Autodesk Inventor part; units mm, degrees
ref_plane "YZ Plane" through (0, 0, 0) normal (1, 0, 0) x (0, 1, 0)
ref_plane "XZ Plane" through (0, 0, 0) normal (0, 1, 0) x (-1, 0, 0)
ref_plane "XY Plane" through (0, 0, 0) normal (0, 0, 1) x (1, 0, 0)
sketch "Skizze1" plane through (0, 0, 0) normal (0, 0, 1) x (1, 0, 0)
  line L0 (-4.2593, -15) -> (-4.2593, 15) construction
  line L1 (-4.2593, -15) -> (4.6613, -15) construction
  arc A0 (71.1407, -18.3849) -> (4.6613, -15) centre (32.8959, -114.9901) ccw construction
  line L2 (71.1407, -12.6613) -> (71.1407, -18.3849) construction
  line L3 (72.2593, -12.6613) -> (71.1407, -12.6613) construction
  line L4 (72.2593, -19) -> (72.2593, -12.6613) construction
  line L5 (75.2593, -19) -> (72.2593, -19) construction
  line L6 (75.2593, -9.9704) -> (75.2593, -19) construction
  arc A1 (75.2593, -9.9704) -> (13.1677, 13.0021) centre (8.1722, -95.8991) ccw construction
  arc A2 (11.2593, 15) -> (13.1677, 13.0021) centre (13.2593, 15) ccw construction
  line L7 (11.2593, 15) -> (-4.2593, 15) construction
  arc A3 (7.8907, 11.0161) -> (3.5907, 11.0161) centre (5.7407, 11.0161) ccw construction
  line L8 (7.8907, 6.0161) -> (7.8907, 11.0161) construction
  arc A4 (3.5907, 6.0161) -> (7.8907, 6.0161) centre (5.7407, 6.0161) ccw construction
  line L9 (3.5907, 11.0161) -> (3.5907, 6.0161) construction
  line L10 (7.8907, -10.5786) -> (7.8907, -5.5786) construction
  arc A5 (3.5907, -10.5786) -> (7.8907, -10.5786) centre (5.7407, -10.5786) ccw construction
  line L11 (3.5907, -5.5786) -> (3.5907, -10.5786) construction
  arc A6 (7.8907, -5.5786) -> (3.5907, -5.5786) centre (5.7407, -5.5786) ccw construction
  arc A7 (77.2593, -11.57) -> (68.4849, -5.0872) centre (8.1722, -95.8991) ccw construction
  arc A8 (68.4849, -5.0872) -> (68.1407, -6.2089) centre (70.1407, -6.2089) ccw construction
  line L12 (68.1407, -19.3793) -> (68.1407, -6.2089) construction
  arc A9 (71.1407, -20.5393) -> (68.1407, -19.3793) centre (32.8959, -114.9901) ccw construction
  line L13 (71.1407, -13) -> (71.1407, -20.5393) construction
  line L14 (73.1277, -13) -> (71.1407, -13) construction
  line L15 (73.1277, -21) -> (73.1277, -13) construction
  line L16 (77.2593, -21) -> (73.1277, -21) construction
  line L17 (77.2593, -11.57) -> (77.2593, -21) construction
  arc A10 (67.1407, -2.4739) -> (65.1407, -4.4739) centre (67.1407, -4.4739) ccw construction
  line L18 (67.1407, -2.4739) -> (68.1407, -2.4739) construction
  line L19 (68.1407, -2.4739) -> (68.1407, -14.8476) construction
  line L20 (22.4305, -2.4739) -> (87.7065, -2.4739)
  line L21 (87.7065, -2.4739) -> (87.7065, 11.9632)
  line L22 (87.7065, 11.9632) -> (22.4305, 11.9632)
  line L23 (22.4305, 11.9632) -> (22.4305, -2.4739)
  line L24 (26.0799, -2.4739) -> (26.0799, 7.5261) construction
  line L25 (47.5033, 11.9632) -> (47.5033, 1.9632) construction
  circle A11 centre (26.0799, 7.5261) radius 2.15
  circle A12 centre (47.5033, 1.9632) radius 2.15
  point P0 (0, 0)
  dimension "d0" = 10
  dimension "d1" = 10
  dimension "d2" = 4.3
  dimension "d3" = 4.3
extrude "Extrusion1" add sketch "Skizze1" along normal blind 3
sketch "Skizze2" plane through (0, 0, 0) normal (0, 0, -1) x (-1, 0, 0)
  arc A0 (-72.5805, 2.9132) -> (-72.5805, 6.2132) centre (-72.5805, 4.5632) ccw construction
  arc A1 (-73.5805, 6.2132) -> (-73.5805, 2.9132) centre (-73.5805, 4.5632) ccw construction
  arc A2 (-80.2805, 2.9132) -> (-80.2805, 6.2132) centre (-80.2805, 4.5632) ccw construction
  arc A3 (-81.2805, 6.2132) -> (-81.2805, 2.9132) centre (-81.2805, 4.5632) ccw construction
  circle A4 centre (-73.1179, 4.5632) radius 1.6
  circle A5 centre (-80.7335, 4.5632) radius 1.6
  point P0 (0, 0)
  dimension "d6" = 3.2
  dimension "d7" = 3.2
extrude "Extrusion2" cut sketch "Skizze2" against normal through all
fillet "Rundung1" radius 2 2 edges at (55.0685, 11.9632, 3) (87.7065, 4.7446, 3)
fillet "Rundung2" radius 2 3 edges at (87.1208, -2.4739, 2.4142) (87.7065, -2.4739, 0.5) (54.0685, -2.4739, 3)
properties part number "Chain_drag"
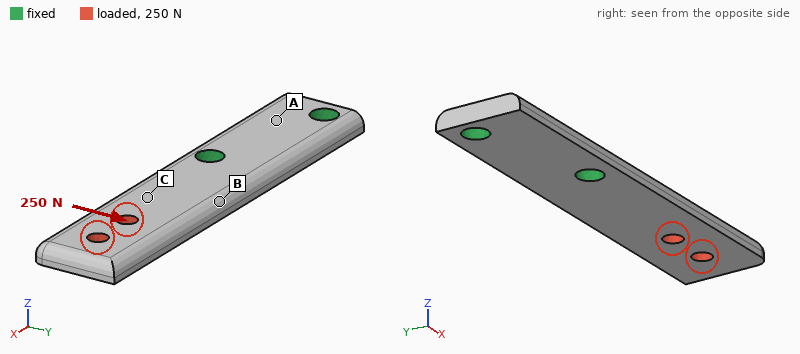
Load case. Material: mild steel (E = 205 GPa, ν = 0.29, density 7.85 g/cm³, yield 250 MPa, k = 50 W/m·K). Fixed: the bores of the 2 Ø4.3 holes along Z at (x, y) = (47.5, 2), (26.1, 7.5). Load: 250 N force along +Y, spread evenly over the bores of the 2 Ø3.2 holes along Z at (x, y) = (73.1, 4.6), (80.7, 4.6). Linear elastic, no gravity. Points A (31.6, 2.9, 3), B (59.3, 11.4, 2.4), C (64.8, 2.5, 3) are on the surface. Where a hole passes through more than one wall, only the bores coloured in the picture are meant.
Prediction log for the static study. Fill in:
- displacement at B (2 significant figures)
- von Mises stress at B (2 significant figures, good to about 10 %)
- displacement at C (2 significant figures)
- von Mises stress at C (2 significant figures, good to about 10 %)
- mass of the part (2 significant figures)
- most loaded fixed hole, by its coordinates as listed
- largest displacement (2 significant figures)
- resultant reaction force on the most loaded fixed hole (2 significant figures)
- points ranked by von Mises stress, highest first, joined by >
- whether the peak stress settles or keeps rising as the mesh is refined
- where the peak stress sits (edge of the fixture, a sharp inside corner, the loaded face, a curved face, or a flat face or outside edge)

8.5 µm
44 MPa
11 µm
16 MPa
20 g
(47.5, 2)
36 µm
450 N
B > C > A
keeps rising
edge of the fixture
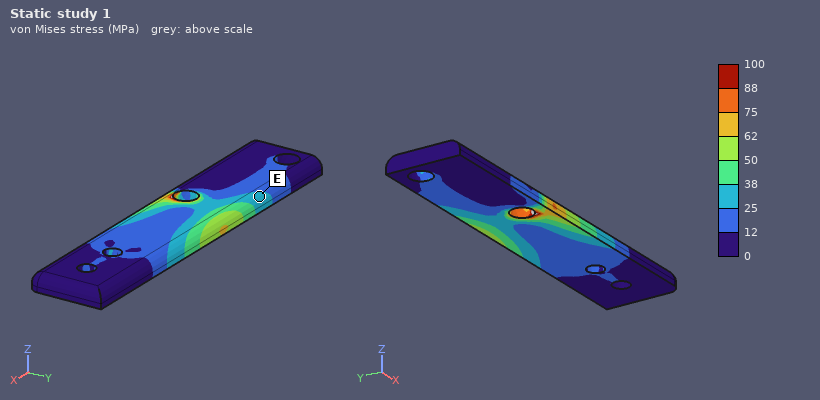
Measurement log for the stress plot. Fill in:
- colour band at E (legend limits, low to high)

25 to 38 MPa
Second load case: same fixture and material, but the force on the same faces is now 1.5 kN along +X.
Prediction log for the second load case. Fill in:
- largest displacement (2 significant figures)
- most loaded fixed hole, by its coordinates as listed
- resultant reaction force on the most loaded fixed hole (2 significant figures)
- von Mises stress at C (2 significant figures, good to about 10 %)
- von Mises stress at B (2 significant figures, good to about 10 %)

11 µm
(47.5, 2)
1.3 kN
40 MPa
35 MPa
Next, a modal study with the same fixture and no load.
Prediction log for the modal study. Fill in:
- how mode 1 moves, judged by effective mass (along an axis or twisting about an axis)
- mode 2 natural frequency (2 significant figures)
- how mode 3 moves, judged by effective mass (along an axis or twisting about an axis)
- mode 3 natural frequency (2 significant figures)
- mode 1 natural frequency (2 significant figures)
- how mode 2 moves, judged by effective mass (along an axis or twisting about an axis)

along Z
5900 Hz
twisting about X
7900 Hz
1600 Hz
along Y
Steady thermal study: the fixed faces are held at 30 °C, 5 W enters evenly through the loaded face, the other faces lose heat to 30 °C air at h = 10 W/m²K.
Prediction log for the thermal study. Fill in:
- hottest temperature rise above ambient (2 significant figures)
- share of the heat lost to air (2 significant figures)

69 K
11 %
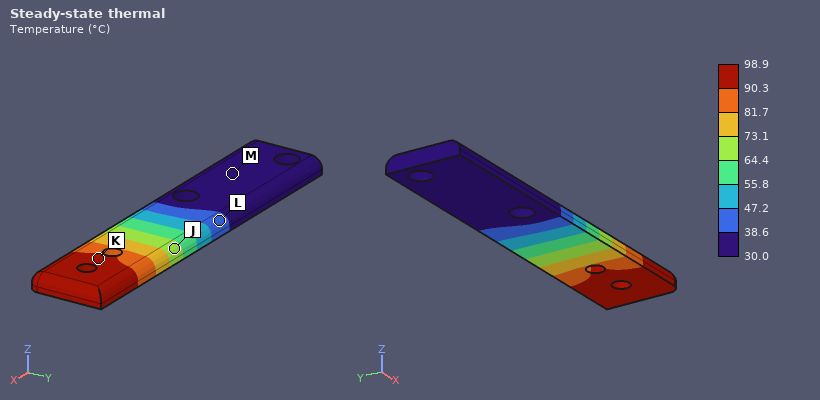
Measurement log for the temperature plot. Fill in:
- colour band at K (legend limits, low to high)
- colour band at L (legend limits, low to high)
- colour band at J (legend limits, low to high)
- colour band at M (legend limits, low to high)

90.3 to 98.9 °C
38.6 to 47.2 °C
64.4 to 73.1 °C
30.0 to 38.6 °C
